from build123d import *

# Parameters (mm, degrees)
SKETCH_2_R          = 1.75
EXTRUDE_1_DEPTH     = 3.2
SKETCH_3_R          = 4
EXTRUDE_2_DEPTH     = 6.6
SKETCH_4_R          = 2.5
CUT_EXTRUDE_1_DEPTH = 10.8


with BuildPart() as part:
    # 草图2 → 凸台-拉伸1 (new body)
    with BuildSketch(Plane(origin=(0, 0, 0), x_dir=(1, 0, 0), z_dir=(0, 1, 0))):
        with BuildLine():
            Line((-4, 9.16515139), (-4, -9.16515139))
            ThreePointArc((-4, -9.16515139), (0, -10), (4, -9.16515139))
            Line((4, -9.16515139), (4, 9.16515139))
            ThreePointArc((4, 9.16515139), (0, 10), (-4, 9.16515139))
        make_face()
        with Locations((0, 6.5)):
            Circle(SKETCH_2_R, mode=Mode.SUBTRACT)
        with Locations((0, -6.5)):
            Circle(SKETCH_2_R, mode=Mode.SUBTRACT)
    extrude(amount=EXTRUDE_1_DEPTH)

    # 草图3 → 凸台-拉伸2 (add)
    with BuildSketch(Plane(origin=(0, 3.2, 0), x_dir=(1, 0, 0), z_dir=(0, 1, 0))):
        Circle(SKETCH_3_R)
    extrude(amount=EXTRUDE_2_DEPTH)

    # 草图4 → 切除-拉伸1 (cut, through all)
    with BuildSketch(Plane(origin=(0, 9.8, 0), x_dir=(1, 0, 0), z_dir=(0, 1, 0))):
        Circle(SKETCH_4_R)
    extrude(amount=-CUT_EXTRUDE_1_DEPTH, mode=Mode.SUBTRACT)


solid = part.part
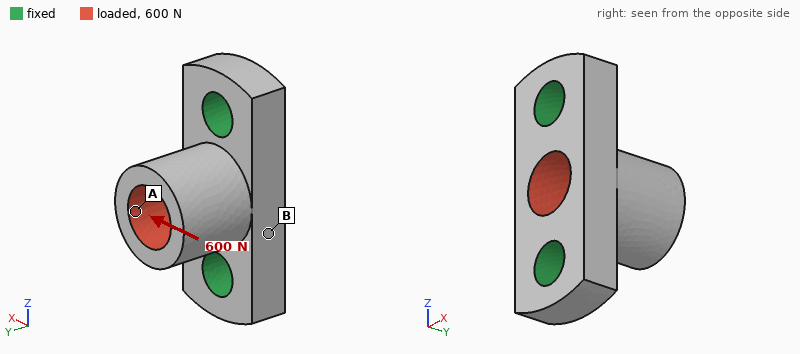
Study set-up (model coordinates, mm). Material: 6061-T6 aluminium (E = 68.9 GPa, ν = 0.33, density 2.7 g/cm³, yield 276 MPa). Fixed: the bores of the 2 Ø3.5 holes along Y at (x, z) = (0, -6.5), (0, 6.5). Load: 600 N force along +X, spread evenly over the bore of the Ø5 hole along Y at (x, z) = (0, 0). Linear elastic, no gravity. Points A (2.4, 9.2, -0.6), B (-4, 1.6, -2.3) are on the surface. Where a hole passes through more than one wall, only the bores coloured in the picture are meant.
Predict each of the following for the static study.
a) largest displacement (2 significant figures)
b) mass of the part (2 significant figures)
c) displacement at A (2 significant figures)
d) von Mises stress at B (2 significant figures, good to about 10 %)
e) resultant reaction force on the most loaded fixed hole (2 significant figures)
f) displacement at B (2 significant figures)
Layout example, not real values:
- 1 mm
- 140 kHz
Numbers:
- 20 µm
- 1.6 g
- 18 µm
- 38 MPa
- 300 N
- 5.4 µm
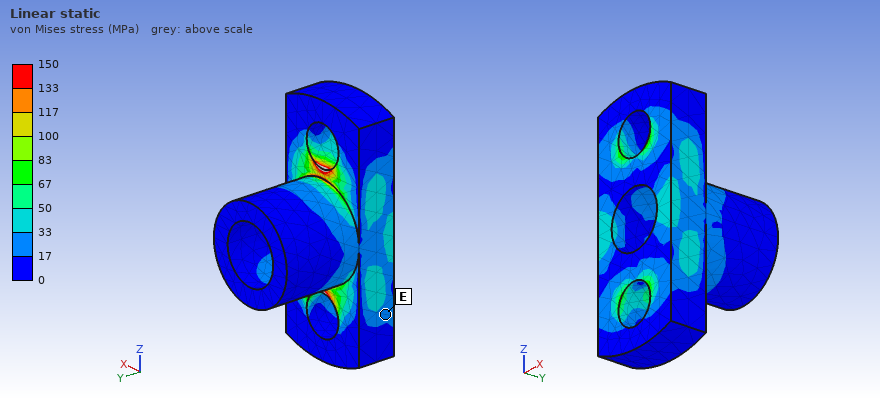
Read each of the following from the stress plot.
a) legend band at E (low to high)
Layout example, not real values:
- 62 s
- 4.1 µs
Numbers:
- 17 to 33 MPa
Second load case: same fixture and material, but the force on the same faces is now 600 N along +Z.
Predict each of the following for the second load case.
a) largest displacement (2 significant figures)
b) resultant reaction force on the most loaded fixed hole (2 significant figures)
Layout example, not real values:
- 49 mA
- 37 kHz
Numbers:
- 7.5 µm
- 360 N
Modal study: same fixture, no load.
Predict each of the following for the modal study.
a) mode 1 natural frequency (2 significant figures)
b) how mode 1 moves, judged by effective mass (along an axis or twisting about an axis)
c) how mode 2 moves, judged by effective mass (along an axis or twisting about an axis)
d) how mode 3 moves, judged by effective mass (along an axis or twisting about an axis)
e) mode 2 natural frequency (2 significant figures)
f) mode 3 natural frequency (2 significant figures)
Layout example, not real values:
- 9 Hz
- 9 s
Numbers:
- 35 kHz
- along X
- along Z
- along Y
- 59 kHz
- 76 kHz
